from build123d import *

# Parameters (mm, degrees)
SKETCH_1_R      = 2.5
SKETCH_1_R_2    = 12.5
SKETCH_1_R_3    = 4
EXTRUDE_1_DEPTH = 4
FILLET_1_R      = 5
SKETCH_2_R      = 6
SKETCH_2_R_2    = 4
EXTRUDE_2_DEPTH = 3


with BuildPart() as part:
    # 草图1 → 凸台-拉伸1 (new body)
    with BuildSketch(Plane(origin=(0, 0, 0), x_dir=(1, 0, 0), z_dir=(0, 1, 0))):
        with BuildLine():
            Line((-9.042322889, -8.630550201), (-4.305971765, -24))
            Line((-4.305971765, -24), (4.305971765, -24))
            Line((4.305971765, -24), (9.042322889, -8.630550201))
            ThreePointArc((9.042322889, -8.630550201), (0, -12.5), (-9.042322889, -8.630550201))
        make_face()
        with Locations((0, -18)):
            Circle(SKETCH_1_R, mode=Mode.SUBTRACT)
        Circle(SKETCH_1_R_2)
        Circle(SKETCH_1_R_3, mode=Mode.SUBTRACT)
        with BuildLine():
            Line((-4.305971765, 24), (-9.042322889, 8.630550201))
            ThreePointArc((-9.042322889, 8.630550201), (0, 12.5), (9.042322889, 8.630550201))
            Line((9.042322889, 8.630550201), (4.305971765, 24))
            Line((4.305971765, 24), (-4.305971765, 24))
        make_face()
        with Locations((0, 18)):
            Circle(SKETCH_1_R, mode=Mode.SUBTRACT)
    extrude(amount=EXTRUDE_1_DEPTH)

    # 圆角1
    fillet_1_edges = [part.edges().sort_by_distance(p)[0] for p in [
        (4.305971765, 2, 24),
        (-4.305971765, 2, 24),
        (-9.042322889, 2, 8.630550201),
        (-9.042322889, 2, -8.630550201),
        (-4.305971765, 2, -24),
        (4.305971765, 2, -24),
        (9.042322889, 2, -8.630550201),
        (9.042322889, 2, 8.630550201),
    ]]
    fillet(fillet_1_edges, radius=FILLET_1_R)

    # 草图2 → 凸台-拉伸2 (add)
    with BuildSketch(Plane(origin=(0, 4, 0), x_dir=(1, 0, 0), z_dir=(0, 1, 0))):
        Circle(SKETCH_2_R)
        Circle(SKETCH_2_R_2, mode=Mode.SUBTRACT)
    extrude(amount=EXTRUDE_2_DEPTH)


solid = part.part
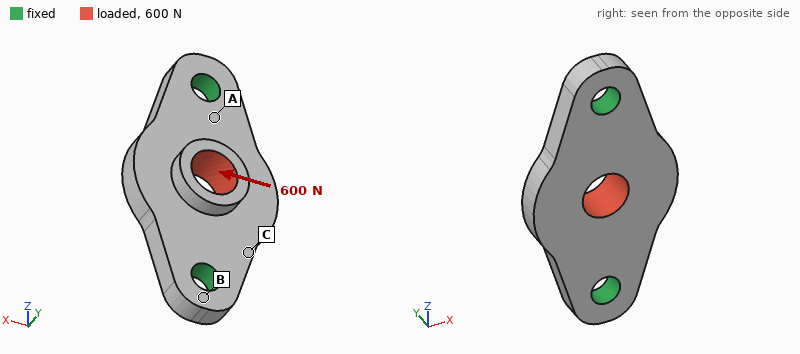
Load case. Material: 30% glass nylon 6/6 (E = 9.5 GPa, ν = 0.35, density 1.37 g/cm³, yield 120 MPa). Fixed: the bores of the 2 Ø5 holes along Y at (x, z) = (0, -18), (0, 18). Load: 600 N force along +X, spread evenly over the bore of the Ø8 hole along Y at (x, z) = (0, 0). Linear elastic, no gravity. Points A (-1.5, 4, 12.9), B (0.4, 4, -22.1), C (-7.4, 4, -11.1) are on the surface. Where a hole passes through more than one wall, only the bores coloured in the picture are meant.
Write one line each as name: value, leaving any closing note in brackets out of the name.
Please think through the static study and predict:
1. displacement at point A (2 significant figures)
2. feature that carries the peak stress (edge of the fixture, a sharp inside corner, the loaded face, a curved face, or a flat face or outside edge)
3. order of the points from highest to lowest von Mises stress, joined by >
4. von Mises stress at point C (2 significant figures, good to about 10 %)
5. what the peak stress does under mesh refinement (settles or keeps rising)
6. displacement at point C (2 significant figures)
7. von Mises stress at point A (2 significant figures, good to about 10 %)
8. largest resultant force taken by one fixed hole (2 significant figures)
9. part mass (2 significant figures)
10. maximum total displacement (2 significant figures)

displacement at point A: 13 µm
feature that carries the peak stress: edge of the fixture
order of the points from highest to lowest von Mises stress, joined by >: A > C > B
von Mises stress at point C: 11 MPa
what the peak stress does under mesh refinement: keeps rising
displacement at point C: 28 µm
von Mises stress at point A: 19 MPa
largest resultant force taken by one fixed hole: 300 N
part mass: 4.1 g
maximum total displacement: 63 µm
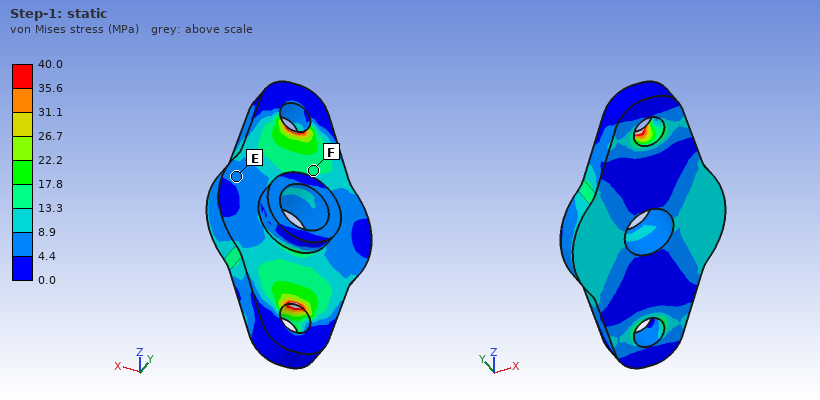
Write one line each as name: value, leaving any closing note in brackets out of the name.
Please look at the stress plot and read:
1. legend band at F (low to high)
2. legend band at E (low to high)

legend band at F: 13.3 to 17.8 MPa
legend band at E: 4.4 to 8.9 MPa
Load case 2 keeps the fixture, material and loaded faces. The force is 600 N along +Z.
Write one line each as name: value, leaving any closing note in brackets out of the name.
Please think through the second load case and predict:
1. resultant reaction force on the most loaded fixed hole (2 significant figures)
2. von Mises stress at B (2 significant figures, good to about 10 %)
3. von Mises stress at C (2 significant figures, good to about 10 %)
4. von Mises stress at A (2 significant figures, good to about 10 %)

resultant reaction force on the most loaded fixed hole: 300 N
von Mises stress at B: 1.5 MPa
von Mises stress at C: 4.1 MPa
von Mises stress at A: 7.1 MPa
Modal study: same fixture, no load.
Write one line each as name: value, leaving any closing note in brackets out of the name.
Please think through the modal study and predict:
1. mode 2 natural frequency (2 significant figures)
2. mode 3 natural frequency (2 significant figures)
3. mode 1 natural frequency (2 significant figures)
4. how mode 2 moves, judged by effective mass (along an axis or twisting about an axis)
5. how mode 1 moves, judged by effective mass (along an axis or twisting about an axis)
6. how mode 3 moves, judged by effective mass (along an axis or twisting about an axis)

mode 2 natural frequency: 7300 Hz
mode 3 natural frequency: 16 kHz
mode 1 natural frequency: 7000 Hz
how mode 2 moves, judged by effective mass: along Y
how mode 1 moves, judged by effective mass: twisting about Z
how mode 3 moves, judged by effective mass: along X
